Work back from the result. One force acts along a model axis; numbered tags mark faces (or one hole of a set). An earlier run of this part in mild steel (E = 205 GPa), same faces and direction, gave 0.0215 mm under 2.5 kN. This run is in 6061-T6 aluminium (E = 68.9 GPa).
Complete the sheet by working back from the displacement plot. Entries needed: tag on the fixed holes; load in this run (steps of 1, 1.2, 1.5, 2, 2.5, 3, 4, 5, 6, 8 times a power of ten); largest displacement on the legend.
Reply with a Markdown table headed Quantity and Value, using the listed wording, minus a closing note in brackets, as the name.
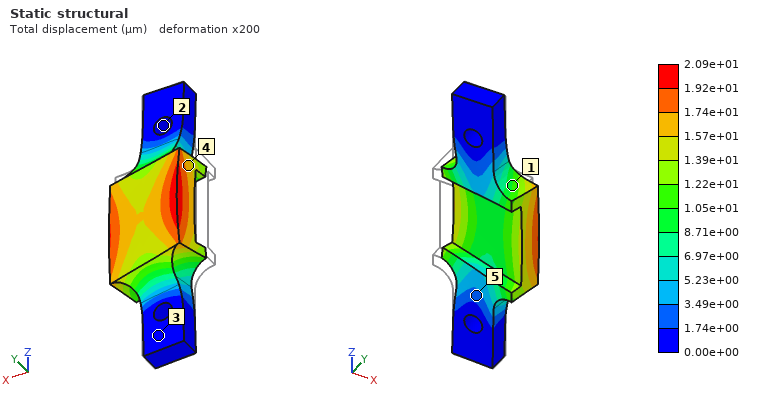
| Quantity | Value |
|---|---|
| tag on the fixed holes | 2 |
| load in this run | 800 N |
| largest displacement on the legend | 2.09e+01 µm |
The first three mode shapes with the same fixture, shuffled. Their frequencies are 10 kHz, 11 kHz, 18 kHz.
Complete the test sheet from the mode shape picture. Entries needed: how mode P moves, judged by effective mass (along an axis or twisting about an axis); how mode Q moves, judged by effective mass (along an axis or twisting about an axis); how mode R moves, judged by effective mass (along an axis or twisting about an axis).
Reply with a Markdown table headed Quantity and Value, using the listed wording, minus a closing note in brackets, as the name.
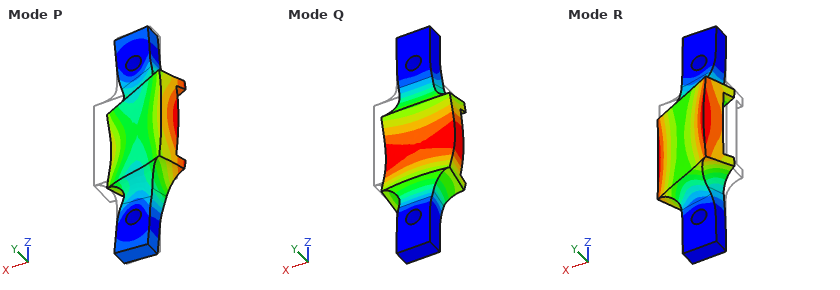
| Quantity | Value |
|---|---|
| how mode P moves, judged by effective mass | along X |
| how mode Q moves, judged by effective mass | along Y |
| how mode R moves, judged by effective mass | along X |
